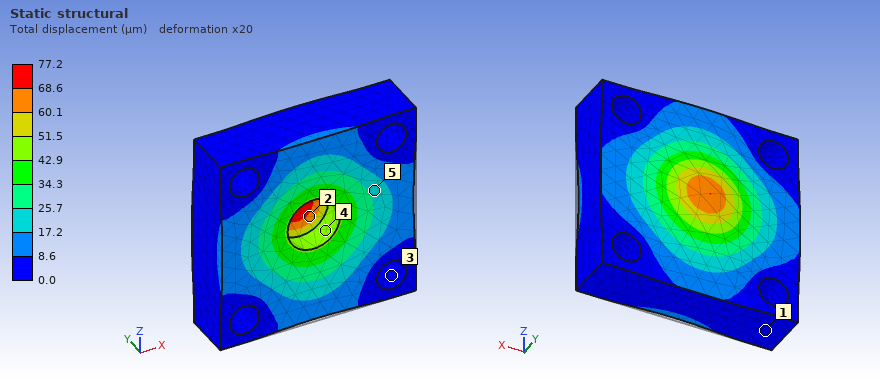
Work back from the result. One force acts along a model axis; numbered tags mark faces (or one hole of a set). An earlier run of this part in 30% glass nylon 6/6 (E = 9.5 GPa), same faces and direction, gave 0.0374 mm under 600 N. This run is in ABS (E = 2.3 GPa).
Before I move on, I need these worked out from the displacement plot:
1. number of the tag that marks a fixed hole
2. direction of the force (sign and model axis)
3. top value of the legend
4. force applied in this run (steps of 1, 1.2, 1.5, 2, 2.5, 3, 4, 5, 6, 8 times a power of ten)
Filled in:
3
+Y
77.2 µm
300 N
